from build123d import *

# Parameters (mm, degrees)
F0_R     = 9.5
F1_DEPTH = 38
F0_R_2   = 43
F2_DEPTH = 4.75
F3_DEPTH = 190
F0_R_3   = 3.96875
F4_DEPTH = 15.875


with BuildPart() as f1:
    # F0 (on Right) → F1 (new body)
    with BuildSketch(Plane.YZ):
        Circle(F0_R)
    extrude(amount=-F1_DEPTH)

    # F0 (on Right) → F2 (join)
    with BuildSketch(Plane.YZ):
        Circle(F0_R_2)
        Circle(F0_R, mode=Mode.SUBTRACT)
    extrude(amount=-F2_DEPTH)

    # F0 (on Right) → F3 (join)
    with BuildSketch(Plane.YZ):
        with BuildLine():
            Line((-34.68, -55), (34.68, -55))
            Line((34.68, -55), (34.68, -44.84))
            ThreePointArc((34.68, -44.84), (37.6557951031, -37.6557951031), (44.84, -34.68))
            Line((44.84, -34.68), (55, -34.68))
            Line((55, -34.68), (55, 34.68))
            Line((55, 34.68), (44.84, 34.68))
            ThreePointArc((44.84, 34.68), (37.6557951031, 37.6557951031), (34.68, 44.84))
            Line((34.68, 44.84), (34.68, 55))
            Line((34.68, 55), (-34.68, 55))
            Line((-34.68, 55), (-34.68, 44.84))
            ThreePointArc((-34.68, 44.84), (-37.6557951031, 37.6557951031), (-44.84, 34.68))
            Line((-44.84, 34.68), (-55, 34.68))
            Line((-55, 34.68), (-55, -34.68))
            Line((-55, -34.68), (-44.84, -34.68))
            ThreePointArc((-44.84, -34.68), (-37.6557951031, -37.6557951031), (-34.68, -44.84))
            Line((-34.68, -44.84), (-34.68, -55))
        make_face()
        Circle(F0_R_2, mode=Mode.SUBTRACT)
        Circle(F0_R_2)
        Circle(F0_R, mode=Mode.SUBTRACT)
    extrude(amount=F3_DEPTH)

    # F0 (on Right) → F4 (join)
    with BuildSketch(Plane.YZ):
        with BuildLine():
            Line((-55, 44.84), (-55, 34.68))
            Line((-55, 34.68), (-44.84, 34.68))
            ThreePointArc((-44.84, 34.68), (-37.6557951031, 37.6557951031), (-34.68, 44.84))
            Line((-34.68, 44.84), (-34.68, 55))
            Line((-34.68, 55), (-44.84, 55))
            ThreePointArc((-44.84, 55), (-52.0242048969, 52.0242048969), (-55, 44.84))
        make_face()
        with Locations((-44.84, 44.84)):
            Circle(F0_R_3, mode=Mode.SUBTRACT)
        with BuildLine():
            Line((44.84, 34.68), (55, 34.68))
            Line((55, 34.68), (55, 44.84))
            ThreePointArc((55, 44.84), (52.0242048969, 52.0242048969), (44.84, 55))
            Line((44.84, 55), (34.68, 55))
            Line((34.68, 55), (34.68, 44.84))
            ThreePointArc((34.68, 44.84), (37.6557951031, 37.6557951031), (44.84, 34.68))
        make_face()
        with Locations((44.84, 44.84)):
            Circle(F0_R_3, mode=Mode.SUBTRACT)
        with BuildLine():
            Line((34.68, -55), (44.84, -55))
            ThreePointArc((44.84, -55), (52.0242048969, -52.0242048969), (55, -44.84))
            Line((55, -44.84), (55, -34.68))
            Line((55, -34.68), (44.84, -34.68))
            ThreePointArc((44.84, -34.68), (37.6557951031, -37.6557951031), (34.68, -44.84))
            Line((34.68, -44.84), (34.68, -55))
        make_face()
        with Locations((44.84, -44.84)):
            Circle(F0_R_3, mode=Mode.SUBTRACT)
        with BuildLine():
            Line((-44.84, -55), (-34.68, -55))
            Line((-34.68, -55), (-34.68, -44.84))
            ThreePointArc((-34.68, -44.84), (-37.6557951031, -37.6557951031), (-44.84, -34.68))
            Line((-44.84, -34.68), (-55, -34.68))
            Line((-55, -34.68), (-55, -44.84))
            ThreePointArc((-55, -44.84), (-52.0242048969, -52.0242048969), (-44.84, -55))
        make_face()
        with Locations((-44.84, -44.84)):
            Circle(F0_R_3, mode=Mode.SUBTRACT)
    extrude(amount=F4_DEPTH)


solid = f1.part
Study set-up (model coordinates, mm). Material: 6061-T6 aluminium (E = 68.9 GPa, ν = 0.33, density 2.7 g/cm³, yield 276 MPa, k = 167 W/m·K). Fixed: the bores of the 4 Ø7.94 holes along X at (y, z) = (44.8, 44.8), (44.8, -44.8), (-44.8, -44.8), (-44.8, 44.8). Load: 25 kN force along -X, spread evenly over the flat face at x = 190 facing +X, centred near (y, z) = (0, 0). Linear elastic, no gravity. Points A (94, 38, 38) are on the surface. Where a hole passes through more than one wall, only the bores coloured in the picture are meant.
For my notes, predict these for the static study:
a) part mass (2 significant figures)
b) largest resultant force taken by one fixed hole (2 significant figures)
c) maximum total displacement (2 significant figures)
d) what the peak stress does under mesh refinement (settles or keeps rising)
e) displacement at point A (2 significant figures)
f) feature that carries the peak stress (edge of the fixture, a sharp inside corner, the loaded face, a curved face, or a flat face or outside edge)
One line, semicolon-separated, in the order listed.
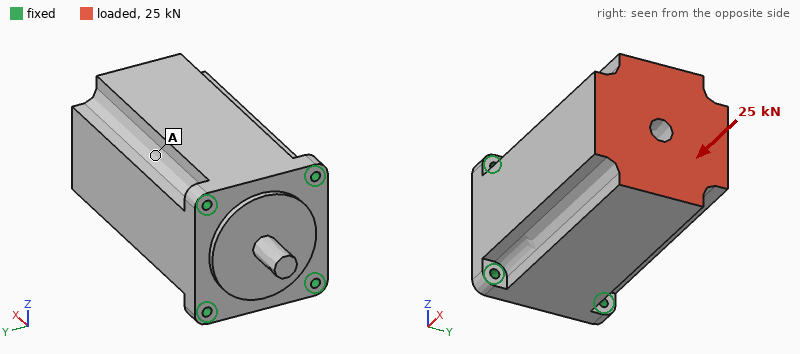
5.4 kg; 6.5 kN; 16 µm; keeps rising; 12 µm; edge of the fixture
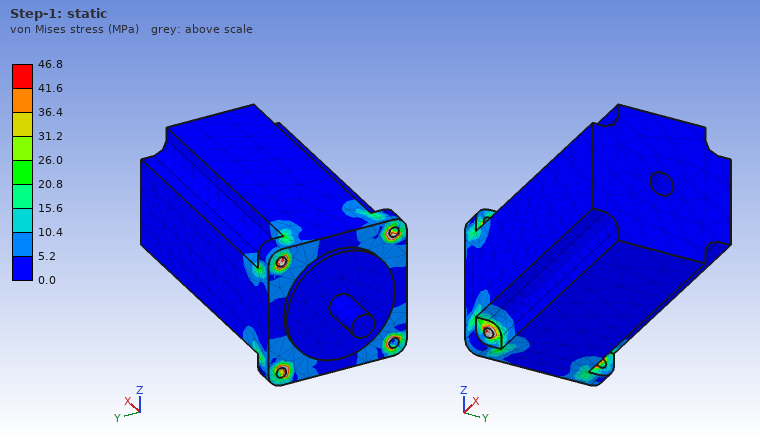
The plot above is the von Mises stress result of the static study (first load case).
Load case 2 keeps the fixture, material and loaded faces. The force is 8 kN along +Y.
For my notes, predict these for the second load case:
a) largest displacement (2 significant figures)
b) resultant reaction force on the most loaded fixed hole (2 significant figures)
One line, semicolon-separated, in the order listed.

88 µm; 8.9 kN
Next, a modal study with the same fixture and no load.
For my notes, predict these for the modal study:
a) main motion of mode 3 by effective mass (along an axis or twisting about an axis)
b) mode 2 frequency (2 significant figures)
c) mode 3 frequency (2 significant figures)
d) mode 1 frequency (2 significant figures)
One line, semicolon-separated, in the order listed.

along X; 1200 Hz; 3200 Hz; 1200 Hz
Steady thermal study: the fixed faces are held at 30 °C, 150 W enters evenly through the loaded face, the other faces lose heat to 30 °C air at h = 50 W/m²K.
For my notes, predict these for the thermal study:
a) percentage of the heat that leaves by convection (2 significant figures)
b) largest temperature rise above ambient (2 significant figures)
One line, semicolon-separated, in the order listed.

33 %; 17 K
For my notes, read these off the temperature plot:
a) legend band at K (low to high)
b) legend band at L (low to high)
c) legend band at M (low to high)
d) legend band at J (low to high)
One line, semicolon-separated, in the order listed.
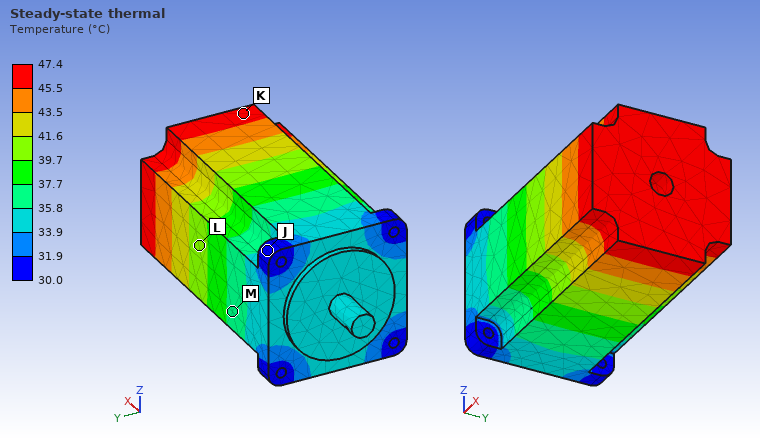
45.5 to 47.4 °C; 39.7 to 41.6 °C; 35.8 to 37.7 °C; 30.0 to 31.9 °C
